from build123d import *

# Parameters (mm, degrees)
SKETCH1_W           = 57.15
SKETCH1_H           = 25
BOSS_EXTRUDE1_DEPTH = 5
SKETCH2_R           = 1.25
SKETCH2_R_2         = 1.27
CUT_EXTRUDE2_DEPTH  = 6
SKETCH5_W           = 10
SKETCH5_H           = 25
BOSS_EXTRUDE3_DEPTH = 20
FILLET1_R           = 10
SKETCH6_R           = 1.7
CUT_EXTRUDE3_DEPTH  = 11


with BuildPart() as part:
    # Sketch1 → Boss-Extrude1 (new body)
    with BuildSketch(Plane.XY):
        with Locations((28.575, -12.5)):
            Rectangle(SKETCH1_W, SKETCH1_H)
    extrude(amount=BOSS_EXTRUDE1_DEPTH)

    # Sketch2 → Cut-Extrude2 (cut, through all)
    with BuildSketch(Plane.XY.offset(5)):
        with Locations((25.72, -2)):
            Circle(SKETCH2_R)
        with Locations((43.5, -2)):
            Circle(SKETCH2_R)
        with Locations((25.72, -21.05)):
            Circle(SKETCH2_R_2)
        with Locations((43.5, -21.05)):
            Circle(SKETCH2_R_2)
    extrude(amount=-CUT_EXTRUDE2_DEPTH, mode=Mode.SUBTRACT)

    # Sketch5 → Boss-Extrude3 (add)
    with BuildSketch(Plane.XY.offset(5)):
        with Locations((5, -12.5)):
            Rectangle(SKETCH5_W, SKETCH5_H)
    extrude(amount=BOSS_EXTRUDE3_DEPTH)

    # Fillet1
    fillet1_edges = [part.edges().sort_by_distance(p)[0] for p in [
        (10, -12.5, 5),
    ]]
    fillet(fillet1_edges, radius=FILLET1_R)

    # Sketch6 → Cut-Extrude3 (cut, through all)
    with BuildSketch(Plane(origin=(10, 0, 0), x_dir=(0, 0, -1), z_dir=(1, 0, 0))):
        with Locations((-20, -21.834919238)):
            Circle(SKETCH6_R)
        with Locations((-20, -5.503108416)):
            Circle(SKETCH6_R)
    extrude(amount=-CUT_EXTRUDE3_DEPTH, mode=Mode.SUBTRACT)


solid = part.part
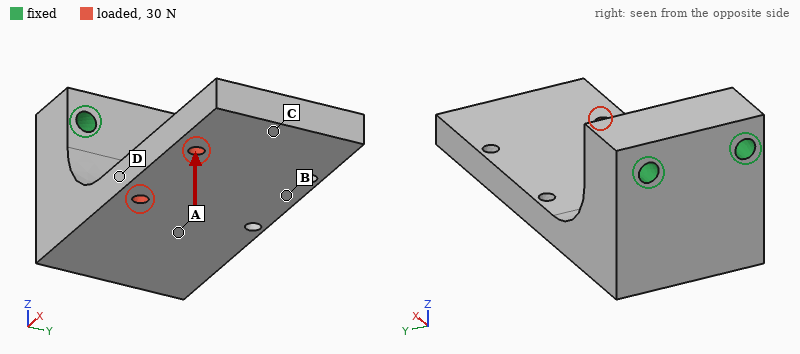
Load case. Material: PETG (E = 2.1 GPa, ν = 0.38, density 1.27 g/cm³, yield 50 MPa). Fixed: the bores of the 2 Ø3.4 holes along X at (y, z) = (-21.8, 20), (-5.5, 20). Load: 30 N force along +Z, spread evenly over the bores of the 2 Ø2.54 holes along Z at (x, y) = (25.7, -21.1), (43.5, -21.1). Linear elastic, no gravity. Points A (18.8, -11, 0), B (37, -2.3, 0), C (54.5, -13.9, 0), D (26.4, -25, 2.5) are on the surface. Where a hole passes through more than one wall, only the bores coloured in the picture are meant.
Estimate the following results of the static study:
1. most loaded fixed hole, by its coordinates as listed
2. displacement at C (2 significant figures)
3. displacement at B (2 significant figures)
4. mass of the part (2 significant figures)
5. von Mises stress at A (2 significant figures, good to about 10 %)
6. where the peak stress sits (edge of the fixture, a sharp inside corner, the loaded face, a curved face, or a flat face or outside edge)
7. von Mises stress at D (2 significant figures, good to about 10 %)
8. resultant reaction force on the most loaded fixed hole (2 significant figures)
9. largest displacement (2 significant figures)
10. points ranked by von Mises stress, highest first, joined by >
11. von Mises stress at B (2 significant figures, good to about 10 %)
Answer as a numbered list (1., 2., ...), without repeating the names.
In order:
1. (-21.8, 20)
2. 0.60 mm
3. 0.25 mm
4. 16 g
5. 4.0 MPa
6. a curved face
7. 2.5 MPa
8. 29 N
9. 0.72 mm
10. A > D > B > C
11. 1.3 MPa
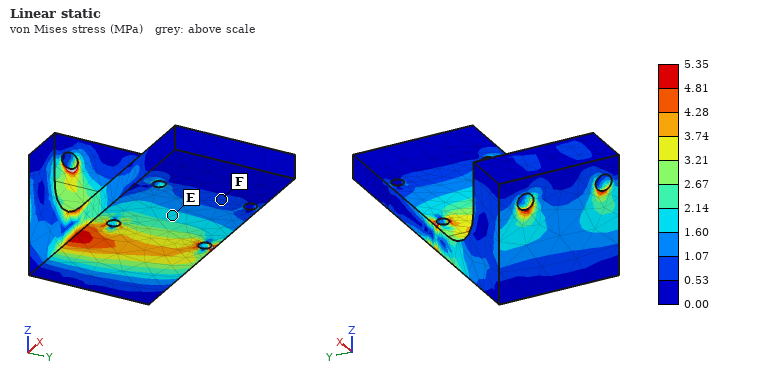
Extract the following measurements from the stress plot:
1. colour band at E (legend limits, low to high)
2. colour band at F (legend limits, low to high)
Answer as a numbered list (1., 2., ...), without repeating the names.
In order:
1. 1.60 to 2.14 MPa
2. 0.53 to 1.07 MPa
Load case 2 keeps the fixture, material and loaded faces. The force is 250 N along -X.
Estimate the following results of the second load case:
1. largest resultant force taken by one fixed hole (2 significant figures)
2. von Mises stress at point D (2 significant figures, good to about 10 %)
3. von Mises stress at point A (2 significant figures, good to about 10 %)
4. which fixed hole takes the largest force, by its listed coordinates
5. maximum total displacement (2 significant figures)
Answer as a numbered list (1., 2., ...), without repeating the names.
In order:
1. 210 N
2. 4.8 MPa
3. 1.9 MPa
4. (-21.8, 20)
5. 0.74 mm
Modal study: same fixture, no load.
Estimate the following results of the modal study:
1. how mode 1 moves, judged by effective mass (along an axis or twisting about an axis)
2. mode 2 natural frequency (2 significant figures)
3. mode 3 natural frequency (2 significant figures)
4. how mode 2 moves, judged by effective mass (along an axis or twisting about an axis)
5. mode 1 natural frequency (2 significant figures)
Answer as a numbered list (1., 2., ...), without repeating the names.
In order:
1. along Z
2. 1100 Hz
3. 1800 Hz
4. along Y
5. 490 Hz
